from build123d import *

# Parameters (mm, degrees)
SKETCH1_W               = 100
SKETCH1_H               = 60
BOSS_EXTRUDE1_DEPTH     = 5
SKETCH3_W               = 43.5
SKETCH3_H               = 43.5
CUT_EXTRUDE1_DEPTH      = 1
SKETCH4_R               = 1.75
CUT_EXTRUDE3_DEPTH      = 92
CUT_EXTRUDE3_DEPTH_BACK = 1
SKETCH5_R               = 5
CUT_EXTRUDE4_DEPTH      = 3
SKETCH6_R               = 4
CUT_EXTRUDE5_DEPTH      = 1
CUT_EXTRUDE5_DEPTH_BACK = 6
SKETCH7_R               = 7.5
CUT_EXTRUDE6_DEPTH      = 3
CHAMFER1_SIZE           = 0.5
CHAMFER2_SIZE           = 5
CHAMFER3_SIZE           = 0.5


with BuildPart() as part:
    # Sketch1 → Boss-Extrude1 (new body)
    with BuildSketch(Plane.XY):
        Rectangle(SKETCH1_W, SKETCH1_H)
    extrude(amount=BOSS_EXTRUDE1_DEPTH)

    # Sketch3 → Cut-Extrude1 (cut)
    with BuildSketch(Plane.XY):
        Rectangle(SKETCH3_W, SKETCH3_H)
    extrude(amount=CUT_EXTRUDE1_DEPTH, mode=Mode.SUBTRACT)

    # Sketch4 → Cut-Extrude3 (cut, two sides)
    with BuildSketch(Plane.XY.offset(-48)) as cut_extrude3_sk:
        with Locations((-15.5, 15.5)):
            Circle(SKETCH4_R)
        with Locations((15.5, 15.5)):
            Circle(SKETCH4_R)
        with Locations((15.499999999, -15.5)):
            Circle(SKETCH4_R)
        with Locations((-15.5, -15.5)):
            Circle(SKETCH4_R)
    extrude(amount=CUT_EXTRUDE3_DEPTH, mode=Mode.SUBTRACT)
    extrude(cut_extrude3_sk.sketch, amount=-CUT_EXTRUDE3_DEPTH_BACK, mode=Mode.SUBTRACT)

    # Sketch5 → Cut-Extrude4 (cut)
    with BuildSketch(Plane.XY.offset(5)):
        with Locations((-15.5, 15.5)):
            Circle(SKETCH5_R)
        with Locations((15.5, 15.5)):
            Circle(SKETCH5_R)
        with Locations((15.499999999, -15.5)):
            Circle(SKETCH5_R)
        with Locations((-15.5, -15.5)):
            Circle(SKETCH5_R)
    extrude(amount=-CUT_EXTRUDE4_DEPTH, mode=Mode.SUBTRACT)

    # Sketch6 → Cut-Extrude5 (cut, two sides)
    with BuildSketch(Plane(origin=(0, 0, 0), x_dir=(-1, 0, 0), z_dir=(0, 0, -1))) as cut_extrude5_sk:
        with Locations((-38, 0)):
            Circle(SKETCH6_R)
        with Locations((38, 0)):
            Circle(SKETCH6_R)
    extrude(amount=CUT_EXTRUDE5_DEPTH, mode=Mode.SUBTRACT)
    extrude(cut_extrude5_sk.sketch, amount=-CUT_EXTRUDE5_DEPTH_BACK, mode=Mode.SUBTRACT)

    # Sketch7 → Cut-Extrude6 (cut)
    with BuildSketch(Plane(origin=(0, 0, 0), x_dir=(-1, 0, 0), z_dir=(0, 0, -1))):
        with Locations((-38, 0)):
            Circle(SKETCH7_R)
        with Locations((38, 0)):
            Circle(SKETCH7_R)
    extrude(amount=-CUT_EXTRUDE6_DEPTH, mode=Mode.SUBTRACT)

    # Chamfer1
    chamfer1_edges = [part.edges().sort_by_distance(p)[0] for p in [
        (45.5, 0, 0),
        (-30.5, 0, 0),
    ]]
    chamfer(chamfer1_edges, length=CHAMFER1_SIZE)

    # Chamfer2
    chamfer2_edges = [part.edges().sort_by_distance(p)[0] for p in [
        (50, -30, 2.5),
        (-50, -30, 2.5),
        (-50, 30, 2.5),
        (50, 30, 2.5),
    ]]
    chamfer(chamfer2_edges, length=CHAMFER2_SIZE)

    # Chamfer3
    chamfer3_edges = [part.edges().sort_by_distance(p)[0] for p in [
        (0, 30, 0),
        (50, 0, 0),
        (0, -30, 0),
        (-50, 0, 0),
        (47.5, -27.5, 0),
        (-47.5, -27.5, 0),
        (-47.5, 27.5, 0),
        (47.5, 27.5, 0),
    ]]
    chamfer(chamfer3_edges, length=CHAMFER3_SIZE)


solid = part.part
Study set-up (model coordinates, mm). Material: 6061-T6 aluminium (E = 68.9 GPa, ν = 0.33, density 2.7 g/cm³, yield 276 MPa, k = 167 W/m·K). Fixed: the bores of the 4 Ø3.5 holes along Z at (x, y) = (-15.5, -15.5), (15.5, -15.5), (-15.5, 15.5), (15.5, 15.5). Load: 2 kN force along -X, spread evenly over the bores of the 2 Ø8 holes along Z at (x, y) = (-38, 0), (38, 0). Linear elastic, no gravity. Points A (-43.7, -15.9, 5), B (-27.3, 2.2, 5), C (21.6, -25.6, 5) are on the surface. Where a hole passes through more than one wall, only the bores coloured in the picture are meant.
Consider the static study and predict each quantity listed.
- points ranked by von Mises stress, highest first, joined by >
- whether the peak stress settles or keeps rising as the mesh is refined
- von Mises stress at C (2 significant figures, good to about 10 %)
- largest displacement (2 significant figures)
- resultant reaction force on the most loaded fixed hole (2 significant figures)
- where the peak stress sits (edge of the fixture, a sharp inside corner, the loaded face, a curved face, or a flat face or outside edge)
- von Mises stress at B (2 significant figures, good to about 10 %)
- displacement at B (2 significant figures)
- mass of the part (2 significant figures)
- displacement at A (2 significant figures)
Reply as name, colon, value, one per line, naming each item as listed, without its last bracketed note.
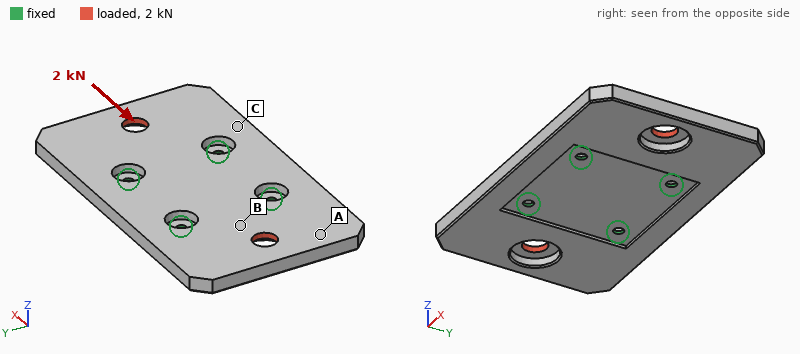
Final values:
points ranked by von Mises stress, highest first, joined by >: B > C > A
whether the peak stress settles or keeps rising as the mesh is refined: keeps rising
von Mises stress at C: 11 MPa
largest displacement: 53 µm
resultant reaction force on the most loaded fixed hole: 510 N
where the peak stress sits: edge of the fixture
von Mises stress at B: 17 MPa
displacement at B: 17 µm
mass of the part: 69 g
displacement at A: 39 µm
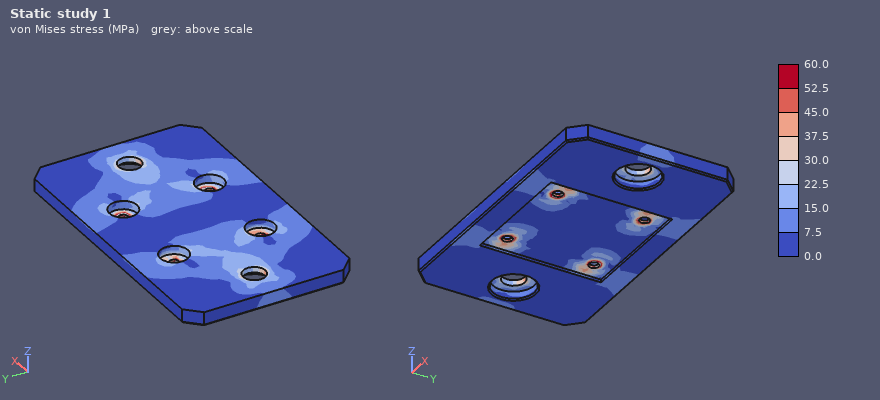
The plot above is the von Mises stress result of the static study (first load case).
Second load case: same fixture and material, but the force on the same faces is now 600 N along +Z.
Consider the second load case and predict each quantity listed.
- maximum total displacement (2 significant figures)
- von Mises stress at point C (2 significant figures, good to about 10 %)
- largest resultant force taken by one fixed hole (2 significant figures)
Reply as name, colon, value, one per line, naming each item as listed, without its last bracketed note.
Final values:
maximum total displacement: 0.19 mm
von Mises stress at point C: 30 MPa
largest resultant force taken by one fixed hole: 580 N
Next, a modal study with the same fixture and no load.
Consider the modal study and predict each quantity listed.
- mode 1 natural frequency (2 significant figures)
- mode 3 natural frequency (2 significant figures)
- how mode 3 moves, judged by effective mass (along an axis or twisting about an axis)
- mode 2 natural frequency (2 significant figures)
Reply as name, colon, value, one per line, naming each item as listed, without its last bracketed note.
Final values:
mode 1 natural frequency: 1900 Hz
mode 3 natural frequency: 3400 Hz
how mode 3 moves, judged by effective mass: twisting about X
mode 2 natural frequency: 1900 Hz
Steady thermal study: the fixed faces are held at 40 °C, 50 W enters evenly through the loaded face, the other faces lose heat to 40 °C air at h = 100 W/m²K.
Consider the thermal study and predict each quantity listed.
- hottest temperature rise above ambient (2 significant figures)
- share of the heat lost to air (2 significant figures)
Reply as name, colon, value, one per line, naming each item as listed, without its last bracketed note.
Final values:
hottest temperature rise above ambient: 31 K
share of the heat lost to air: 36 %
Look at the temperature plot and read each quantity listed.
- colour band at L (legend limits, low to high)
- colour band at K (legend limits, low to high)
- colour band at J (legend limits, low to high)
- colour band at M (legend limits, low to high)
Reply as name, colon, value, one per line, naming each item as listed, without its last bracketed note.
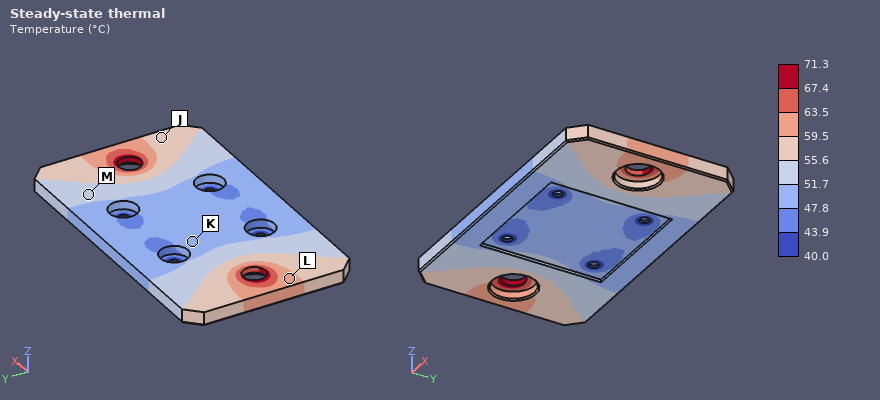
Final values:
colour band at L: 59.5 to 63.5 °C
colour band at K: 47.8 to 51.7 °C
colour band at J: 55.6 to 59.5 °C
colour band at M: 51.7 to 55.6 °C
